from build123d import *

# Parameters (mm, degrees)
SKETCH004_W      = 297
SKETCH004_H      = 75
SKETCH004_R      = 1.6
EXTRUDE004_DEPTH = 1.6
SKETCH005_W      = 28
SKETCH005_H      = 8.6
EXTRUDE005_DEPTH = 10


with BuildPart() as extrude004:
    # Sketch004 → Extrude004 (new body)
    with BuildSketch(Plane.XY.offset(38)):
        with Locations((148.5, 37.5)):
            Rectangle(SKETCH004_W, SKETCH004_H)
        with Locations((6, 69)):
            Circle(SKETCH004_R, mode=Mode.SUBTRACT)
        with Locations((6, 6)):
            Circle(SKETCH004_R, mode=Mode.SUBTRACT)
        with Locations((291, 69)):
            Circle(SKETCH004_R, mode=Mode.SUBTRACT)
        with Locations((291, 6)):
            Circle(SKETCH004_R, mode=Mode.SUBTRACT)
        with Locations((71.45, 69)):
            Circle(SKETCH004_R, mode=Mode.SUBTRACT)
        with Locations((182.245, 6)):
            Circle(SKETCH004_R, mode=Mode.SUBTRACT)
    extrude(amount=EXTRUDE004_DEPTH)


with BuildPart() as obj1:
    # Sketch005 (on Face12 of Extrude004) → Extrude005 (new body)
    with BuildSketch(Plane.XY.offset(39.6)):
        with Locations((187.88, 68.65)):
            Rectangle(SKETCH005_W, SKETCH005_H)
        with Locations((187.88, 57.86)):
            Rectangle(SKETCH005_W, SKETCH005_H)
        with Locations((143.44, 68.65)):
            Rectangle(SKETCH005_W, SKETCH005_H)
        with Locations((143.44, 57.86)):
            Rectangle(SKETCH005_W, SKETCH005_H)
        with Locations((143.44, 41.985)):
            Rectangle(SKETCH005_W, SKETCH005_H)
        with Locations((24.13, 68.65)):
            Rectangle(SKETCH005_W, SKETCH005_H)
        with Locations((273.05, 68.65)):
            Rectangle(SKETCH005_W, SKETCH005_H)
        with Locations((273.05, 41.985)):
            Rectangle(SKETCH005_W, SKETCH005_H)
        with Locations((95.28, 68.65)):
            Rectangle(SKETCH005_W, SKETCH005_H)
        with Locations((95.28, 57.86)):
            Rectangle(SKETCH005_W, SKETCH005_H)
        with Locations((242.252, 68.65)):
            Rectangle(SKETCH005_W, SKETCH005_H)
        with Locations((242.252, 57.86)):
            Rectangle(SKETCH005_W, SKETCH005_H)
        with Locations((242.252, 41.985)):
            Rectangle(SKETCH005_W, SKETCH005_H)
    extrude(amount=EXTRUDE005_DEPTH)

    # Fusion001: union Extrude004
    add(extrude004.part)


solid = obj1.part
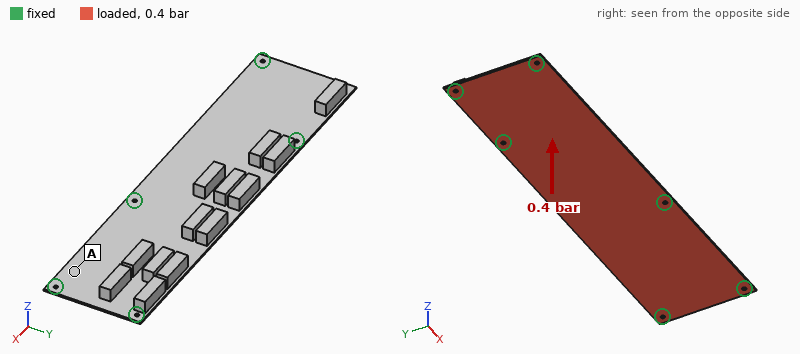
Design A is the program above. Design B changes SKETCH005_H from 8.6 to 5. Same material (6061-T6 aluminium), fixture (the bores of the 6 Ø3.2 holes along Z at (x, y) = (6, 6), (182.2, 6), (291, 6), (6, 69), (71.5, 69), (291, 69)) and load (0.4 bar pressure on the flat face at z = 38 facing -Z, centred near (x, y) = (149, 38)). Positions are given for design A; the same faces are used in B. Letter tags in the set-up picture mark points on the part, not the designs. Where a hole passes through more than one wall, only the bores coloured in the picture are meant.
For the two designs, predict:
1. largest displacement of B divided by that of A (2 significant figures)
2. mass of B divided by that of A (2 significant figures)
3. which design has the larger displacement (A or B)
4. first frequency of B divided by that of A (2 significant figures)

1.1
0.80
B
1.1
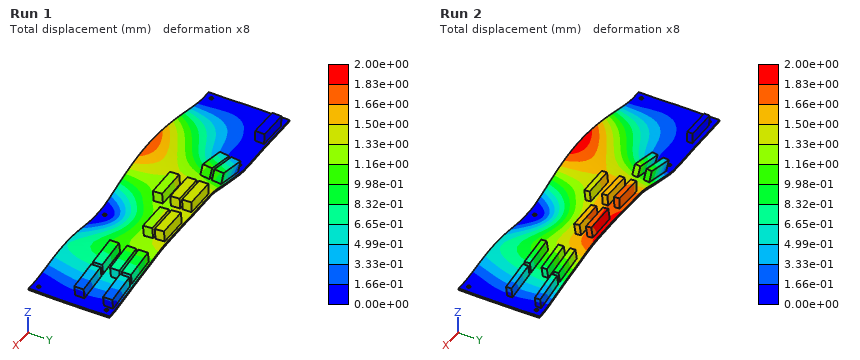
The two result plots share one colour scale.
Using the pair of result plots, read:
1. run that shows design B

Run 2
